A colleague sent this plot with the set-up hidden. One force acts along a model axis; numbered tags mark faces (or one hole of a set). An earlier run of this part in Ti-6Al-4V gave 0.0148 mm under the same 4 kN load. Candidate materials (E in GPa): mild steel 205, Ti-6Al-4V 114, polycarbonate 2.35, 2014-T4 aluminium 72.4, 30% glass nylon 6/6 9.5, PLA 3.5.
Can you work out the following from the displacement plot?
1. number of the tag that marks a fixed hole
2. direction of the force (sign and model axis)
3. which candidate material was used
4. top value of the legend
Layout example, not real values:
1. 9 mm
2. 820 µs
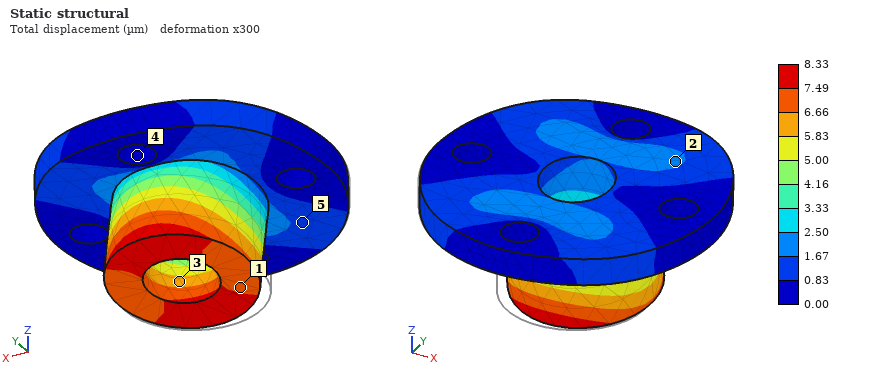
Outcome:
1. 4
2. +Y
3. mild steel
4. 8.33 µm
